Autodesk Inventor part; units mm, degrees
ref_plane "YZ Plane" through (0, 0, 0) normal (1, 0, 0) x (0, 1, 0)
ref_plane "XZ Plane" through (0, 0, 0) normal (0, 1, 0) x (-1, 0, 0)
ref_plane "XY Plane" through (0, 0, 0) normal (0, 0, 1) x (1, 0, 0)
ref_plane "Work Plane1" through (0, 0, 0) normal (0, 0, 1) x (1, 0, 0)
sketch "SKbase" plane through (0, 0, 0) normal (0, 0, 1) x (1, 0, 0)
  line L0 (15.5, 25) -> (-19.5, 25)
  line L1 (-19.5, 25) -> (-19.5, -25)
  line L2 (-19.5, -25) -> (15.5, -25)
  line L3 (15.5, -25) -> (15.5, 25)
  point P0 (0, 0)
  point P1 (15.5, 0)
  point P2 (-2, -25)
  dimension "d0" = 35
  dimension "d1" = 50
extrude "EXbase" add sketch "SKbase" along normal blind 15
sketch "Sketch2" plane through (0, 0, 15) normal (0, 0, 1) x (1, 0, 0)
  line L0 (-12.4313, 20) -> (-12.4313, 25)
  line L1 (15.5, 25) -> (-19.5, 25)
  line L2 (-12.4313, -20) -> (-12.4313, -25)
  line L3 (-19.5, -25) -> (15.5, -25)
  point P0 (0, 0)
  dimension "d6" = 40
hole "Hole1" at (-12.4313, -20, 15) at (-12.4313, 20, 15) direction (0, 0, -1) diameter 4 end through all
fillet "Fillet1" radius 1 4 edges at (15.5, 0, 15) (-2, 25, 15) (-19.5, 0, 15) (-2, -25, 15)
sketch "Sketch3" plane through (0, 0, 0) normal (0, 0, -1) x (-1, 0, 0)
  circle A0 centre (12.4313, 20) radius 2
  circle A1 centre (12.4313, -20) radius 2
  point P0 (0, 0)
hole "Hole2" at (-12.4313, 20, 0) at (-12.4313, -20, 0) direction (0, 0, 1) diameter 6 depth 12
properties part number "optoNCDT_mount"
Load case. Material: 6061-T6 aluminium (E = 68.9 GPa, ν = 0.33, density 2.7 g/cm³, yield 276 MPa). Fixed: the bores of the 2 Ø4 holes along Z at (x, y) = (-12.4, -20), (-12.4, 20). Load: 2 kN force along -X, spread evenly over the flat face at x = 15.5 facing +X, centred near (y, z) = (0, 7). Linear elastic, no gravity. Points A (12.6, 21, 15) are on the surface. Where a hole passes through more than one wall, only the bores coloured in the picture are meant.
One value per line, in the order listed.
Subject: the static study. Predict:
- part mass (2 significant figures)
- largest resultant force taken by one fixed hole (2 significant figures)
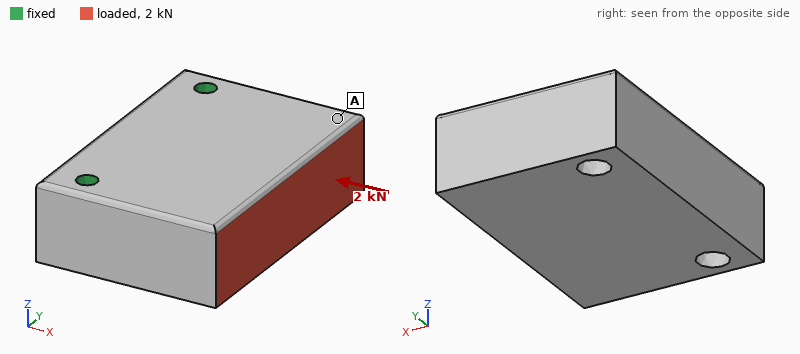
69 g
1.0 kN
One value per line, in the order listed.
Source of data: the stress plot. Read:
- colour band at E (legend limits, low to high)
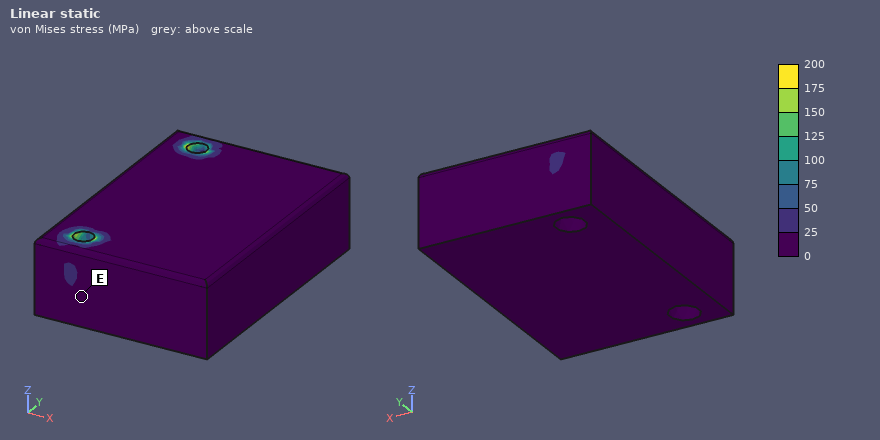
0 to 25 MPa
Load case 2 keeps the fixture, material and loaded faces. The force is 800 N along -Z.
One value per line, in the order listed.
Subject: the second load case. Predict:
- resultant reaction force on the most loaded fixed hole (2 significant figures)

420 N
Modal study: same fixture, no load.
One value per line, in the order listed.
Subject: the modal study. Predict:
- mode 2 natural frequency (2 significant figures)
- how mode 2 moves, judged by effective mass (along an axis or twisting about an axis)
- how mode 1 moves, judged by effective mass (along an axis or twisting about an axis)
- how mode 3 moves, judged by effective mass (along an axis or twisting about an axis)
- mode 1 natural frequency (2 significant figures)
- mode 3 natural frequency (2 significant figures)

12 kHz
along Y
along Z
along Y
2600 Hz
14 kHz
